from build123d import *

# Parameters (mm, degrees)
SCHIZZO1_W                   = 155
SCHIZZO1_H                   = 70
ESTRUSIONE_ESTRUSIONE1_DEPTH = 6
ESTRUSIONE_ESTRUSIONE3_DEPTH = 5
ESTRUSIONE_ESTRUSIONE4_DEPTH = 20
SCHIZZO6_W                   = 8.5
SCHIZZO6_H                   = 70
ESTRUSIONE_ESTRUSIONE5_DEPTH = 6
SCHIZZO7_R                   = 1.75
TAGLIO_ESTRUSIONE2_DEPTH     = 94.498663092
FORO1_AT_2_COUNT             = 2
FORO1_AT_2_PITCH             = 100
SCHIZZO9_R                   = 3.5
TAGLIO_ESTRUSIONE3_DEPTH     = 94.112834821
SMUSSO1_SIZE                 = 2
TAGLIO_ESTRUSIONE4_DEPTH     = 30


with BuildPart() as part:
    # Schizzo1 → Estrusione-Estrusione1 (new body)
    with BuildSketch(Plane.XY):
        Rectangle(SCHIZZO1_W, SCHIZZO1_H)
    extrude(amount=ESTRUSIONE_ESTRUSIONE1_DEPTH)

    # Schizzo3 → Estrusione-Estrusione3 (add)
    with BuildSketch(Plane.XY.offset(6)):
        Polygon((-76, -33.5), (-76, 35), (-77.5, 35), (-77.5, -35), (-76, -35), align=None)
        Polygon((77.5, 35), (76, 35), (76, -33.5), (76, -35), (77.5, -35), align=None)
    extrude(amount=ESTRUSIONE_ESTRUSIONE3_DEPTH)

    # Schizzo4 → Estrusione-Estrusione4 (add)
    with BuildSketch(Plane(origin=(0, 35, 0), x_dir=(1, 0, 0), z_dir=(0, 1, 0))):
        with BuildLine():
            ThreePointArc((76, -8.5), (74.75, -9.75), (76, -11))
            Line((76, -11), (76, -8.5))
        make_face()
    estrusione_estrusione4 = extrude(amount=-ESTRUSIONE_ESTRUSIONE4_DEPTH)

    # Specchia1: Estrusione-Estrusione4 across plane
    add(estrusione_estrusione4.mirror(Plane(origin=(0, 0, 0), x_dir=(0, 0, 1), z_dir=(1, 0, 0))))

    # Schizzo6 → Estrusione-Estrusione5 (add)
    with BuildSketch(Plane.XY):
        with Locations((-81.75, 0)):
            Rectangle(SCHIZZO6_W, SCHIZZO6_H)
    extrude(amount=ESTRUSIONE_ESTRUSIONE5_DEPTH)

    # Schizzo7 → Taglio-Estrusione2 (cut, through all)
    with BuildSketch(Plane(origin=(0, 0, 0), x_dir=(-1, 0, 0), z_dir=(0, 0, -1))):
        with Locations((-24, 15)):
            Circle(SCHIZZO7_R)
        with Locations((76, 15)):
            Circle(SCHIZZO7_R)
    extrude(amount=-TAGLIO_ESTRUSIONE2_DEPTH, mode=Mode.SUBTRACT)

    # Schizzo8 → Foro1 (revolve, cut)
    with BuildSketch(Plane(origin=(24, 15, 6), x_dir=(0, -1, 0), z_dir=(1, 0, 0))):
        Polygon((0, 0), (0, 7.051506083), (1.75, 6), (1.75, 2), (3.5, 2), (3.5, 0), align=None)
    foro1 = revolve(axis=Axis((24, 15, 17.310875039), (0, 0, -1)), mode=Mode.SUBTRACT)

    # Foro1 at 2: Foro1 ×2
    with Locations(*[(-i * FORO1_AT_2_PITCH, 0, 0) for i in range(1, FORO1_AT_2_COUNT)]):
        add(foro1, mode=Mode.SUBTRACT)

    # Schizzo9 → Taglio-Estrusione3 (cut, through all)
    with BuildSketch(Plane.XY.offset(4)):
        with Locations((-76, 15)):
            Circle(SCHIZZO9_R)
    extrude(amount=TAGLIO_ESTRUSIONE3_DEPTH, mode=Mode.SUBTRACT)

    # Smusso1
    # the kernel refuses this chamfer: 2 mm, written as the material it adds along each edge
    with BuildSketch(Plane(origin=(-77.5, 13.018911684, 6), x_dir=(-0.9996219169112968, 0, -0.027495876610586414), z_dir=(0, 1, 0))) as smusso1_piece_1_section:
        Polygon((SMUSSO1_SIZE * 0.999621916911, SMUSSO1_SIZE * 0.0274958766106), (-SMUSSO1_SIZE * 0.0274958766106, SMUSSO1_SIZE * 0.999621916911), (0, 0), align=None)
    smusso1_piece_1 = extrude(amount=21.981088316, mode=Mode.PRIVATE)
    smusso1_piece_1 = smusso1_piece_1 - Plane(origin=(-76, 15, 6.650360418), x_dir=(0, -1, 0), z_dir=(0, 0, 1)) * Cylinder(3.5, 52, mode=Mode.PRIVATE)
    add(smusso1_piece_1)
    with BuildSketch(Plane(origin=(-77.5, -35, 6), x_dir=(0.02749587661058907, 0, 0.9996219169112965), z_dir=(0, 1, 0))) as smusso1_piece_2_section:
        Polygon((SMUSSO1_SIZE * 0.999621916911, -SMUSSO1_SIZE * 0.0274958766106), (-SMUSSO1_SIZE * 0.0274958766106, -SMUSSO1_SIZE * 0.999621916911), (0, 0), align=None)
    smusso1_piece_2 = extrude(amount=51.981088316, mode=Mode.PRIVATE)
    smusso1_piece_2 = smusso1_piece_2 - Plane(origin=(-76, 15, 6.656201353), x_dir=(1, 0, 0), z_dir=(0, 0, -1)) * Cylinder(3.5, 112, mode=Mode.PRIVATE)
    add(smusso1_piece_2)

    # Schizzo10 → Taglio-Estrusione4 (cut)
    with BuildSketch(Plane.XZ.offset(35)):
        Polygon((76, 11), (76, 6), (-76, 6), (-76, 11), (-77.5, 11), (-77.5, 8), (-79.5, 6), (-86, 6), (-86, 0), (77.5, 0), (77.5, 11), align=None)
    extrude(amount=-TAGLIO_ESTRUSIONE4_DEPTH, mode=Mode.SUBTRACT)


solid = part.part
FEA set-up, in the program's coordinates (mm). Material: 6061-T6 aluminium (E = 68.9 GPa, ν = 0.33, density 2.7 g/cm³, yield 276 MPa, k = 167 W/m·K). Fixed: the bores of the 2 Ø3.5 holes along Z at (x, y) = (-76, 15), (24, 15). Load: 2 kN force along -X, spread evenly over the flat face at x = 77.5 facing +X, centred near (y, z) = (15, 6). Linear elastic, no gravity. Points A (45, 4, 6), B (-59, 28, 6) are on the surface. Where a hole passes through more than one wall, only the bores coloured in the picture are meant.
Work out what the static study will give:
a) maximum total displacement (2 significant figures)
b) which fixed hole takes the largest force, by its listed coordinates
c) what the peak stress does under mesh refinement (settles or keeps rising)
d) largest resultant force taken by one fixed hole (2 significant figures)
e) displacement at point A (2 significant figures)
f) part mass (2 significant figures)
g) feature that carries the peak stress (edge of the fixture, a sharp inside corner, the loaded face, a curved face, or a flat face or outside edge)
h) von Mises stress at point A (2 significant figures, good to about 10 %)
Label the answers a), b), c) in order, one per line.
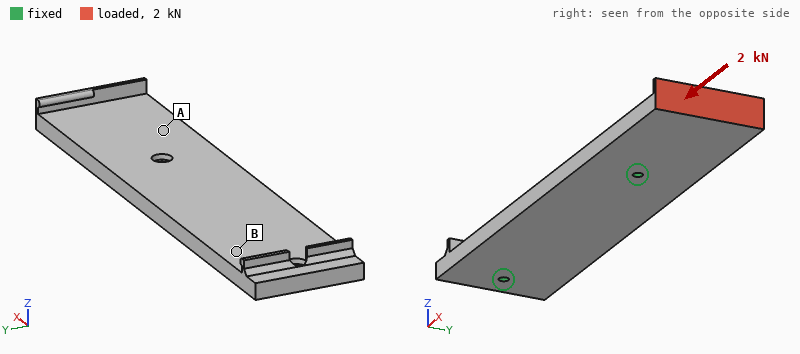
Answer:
a) 0.24 mm
b) (24, 15)
c) keeps rising
d) 1.5 kN
e) 0.052 mm
f) 110 g
g) edge of the fixture
h) 29 MPa
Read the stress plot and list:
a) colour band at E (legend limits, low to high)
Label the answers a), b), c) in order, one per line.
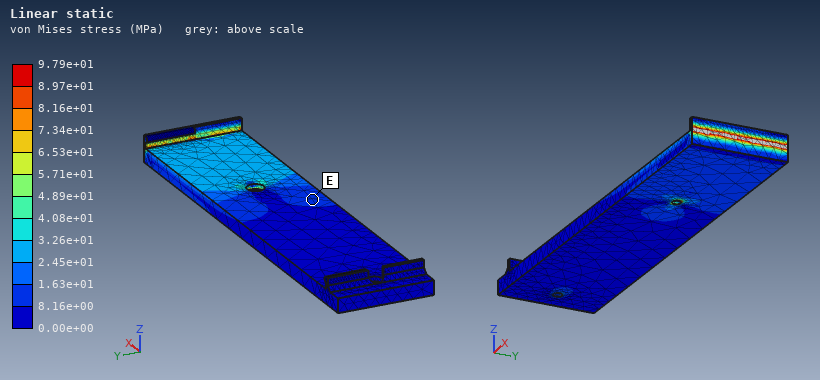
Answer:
a) 8.16e+00 to 1.63e+01 MPa
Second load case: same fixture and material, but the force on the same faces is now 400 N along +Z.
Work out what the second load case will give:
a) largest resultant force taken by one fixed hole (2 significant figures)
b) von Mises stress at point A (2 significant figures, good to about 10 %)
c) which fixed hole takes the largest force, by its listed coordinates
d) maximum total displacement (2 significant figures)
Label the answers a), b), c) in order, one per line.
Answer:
a) 740 N
b) 52 MPa
c) (24, 15)
d) 0.63 mm
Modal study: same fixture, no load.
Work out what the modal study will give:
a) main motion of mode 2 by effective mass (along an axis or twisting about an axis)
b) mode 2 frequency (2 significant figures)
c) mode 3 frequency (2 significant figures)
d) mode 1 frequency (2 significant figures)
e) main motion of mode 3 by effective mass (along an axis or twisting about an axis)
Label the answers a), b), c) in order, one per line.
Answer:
a) along Z
b) 2400 Hz
c) 2700 Hz
d) 1200 Hz
e) twisting about X
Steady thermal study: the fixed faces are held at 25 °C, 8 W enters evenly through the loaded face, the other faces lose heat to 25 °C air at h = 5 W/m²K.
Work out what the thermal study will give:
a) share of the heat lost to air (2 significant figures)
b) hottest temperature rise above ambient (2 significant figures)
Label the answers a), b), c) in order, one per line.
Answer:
a) 3.1 %
b) 14 K
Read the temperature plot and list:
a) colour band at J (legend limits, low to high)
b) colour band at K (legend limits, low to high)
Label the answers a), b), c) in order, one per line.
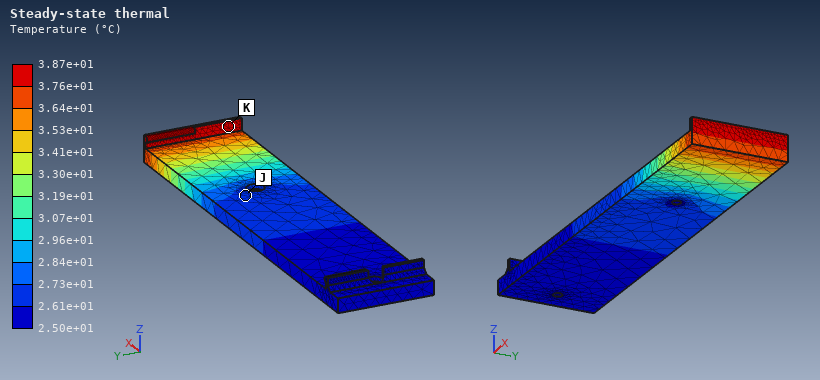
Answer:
a) 2.61e+01 to 2.73e+01 °C
b) 3.76e+01 to 3.87e+01 °C
